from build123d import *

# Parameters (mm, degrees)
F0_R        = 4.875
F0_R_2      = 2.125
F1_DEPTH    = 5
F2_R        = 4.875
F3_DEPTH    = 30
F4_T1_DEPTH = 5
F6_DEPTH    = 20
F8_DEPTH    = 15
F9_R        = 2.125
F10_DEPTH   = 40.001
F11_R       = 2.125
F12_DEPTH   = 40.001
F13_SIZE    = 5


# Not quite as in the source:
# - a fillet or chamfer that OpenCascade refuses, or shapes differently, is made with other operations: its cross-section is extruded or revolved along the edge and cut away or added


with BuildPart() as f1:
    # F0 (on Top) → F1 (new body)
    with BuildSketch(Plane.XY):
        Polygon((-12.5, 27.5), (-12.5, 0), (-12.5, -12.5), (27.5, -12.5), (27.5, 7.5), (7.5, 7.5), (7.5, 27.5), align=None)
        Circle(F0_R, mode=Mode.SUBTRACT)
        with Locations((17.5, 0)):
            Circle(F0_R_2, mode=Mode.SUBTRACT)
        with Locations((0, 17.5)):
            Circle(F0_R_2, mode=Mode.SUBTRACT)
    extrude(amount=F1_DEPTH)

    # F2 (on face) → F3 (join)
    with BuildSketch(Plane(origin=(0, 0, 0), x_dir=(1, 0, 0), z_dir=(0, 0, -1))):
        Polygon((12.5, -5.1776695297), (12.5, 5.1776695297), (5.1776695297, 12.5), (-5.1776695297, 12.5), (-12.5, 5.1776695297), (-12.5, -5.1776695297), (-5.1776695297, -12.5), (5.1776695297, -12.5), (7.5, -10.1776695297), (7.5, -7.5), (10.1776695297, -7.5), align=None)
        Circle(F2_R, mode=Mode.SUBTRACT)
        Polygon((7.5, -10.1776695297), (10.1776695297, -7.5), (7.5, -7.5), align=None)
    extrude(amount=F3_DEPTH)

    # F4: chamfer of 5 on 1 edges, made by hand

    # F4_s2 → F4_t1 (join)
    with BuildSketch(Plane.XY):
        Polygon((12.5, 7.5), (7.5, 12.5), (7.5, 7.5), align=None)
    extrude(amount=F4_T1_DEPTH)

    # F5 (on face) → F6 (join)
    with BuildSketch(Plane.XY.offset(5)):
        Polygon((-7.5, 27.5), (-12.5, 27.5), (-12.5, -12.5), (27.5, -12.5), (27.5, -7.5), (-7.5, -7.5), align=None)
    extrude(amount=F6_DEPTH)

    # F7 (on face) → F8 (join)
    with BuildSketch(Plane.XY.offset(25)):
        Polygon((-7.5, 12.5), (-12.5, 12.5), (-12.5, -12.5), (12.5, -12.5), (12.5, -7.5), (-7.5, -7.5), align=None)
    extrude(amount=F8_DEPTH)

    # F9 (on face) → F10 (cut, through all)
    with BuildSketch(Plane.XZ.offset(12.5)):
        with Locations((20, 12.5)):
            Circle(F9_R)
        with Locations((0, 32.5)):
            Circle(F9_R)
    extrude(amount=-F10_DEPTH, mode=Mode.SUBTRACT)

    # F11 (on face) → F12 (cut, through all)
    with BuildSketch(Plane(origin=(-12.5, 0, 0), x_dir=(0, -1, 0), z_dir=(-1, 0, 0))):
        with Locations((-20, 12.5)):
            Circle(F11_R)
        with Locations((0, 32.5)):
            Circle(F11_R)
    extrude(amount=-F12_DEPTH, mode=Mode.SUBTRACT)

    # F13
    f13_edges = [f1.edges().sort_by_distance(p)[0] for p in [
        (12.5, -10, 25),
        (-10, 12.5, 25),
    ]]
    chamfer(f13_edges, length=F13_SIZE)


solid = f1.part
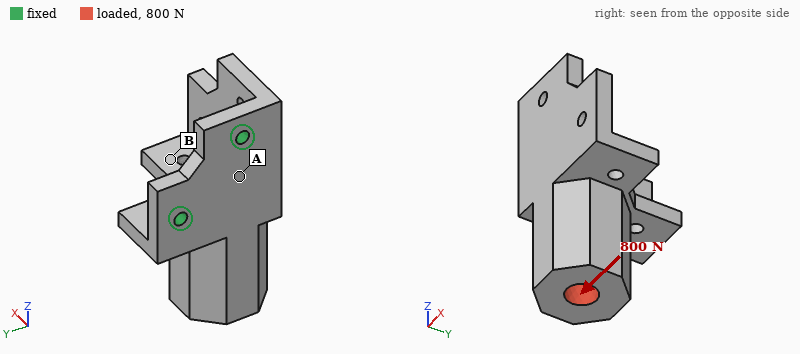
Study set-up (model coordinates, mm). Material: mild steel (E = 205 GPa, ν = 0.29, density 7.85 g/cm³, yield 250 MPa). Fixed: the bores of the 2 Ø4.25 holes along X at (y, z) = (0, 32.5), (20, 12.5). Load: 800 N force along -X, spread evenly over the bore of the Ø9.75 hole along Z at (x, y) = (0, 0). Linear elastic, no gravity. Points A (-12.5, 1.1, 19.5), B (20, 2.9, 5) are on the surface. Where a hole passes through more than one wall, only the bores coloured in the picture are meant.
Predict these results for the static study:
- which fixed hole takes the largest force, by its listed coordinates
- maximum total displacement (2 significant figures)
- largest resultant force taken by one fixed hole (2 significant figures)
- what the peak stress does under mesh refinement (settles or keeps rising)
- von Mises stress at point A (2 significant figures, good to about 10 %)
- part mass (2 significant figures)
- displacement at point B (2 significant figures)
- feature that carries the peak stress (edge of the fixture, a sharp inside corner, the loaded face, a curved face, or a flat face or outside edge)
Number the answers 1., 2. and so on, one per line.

1. (20, 12.5)
2. 0.12 mm
3. 760 N
4. keeps rising
5. 48 MPa
6. 230 g
7. 0.076 mm
8. edge of the fixture
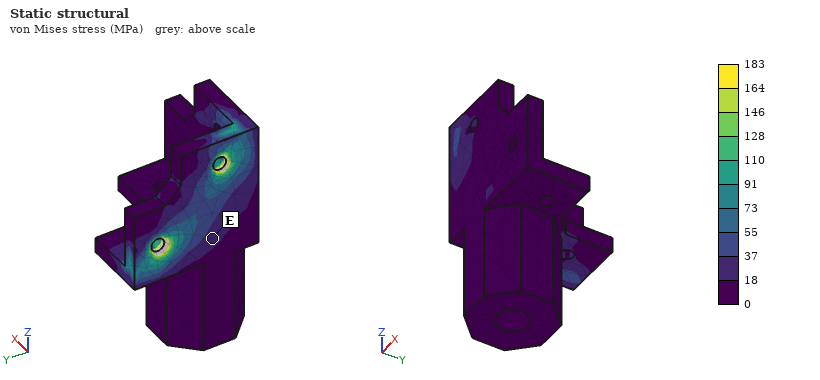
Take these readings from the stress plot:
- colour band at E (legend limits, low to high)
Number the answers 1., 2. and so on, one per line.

1. 18 to 37 MPa
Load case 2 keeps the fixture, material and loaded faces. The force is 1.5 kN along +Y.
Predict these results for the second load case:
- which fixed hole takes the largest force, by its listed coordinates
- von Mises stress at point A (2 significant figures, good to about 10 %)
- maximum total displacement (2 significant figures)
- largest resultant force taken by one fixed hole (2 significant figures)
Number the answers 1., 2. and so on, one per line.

1. (20, 12.5)
2. 29 MPa
3. 57 µm
4. 2.3 kN
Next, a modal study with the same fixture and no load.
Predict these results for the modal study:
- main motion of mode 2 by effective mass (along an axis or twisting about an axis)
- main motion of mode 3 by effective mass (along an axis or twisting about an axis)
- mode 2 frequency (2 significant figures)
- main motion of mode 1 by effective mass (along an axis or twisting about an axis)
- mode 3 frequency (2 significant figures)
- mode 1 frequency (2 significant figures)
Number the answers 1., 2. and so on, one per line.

1. along Y
2. along Y
3. 4200 Hz
4. along X
5. 5400 Hz
6. 1200 Hz
